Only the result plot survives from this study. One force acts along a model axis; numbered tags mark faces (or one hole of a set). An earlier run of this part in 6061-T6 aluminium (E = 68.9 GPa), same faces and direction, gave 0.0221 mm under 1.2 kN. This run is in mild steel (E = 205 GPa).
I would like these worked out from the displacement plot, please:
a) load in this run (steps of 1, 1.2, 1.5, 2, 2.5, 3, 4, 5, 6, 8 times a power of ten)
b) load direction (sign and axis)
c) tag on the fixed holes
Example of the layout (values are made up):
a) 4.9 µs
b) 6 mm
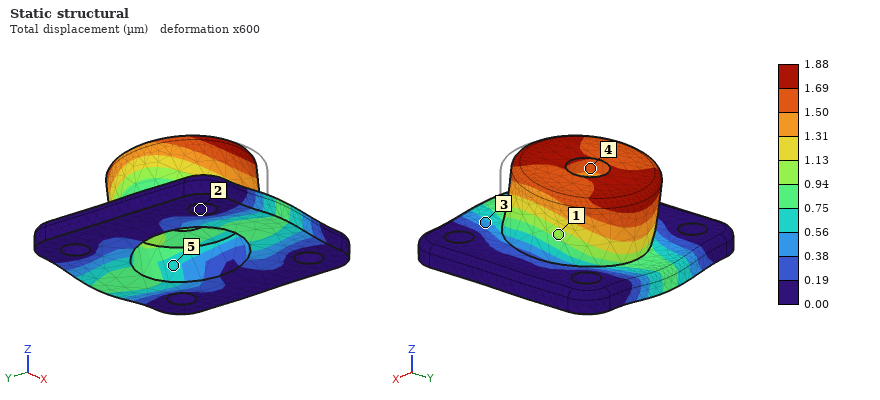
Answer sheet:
a) 300 N
b) +Y
c) 2
